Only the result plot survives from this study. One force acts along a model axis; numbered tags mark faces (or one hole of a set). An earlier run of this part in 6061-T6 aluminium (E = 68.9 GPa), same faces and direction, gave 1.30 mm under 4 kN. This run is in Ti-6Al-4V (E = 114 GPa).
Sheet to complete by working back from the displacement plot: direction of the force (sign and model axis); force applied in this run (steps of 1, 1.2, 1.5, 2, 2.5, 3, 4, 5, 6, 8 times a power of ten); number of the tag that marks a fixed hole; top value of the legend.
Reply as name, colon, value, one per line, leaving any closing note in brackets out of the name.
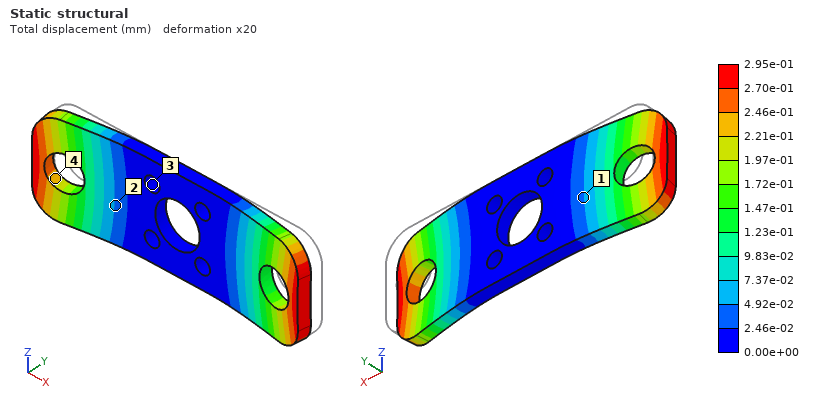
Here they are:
direction of the force: -Y
force applied in this run: 1.5 kN
number of the tag that marks a fixed hole: 3
top value of the legend: 2.95e-01 mm
